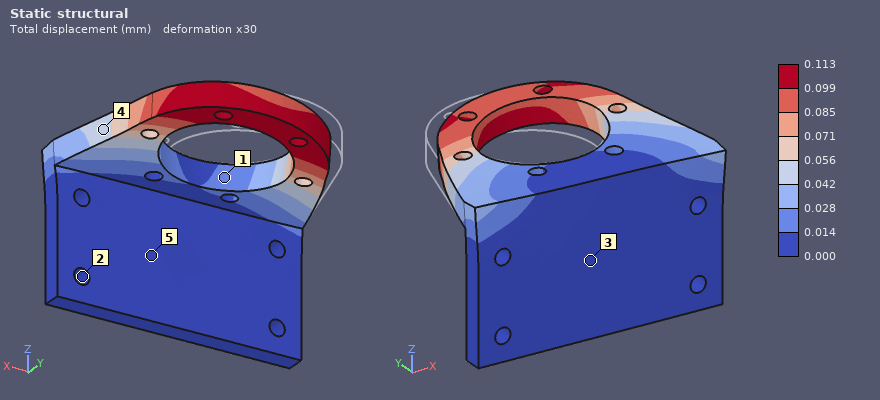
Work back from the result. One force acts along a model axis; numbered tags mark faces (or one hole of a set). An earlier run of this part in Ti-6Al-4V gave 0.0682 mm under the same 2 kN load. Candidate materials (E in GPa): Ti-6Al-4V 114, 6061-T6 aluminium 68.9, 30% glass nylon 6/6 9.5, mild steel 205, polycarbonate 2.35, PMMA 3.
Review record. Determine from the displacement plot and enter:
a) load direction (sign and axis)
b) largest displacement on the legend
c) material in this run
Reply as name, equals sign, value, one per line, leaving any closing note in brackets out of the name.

load direction = +X
largest displacement on the legend = 0.113 mm
material in this run = 6061-T6 aluminium
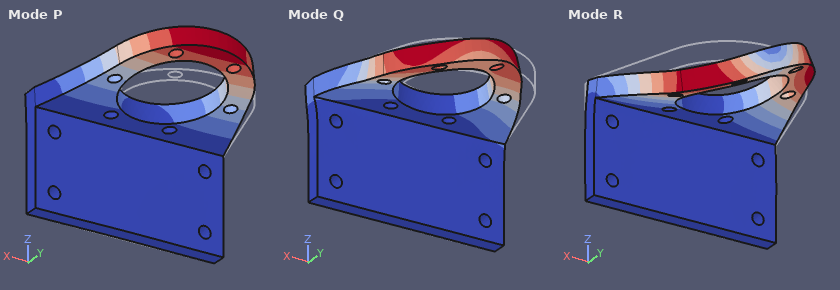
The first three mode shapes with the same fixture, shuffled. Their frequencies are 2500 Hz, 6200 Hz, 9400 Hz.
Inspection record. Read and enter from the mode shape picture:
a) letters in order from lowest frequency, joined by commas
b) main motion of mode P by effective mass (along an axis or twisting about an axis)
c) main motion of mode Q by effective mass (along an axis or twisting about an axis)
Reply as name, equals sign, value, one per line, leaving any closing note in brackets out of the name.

letters in order from lowest frequency, joined by commas = P, R, Q
main motion of mode P by effective mass = along Z
main motion of mode Q by effective mass = along X
